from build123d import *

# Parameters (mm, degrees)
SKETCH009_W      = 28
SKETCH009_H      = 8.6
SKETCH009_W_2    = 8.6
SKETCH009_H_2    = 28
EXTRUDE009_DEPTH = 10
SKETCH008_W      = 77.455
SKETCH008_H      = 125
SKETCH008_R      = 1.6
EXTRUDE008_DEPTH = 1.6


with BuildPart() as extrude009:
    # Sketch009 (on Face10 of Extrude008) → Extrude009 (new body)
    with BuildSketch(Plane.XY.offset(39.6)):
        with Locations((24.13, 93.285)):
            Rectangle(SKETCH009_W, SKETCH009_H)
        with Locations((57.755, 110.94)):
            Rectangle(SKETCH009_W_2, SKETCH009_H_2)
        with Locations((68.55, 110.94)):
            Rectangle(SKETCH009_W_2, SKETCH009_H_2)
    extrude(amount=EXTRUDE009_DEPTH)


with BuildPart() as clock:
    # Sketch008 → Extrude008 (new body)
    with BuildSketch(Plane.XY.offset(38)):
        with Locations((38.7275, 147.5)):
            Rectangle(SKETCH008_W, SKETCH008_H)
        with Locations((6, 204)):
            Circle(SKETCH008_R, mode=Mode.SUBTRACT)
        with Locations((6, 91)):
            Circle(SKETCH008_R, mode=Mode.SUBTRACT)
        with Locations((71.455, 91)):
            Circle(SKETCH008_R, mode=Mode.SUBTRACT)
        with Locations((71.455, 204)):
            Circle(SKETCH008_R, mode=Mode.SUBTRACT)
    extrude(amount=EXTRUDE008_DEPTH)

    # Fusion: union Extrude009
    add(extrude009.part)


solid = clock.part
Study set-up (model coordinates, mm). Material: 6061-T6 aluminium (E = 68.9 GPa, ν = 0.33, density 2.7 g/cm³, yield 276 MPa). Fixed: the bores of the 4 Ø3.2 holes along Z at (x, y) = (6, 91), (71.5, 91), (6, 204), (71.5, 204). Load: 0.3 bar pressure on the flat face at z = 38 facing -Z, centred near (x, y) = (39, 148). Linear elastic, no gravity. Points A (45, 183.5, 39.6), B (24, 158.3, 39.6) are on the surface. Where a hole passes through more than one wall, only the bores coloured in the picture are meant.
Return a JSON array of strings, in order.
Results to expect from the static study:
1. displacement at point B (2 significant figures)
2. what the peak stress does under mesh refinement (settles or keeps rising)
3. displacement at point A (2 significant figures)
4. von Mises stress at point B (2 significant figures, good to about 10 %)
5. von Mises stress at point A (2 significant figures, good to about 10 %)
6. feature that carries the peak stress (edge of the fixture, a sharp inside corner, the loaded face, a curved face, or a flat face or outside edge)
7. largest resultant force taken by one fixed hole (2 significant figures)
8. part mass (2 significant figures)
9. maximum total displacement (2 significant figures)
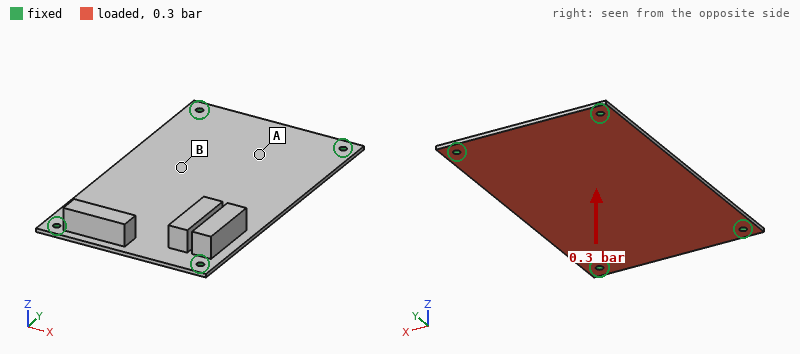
["0.65 mm", "keeps rising", "0.36 mm", "35 MPa", "17 MPa", "edge of the fixture", "80 N", "61 g", "0.69 mm"]
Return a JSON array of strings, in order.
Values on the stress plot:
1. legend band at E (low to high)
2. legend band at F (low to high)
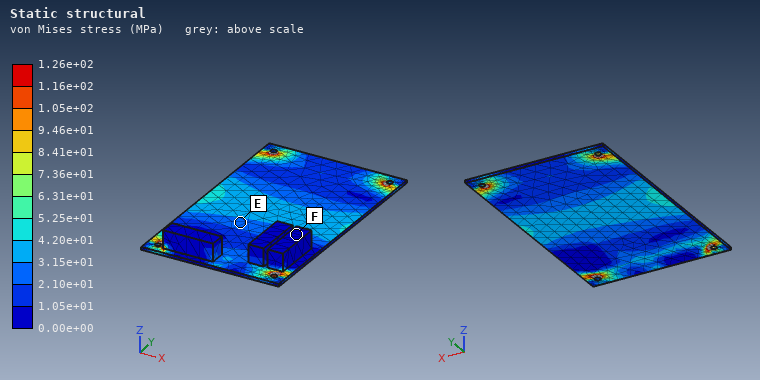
["2.10e+01 to 3.15e+01 MPa", "0.00e+00 to 1.05e+01 MPa"]
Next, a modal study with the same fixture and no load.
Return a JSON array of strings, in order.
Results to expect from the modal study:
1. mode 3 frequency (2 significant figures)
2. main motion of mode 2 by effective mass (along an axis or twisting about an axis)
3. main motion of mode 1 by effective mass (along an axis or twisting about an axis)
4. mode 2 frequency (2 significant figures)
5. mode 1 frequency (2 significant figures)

["1400 Hz", "twisting about Y", "along Z", "970 Hz", "540 Hz"]
